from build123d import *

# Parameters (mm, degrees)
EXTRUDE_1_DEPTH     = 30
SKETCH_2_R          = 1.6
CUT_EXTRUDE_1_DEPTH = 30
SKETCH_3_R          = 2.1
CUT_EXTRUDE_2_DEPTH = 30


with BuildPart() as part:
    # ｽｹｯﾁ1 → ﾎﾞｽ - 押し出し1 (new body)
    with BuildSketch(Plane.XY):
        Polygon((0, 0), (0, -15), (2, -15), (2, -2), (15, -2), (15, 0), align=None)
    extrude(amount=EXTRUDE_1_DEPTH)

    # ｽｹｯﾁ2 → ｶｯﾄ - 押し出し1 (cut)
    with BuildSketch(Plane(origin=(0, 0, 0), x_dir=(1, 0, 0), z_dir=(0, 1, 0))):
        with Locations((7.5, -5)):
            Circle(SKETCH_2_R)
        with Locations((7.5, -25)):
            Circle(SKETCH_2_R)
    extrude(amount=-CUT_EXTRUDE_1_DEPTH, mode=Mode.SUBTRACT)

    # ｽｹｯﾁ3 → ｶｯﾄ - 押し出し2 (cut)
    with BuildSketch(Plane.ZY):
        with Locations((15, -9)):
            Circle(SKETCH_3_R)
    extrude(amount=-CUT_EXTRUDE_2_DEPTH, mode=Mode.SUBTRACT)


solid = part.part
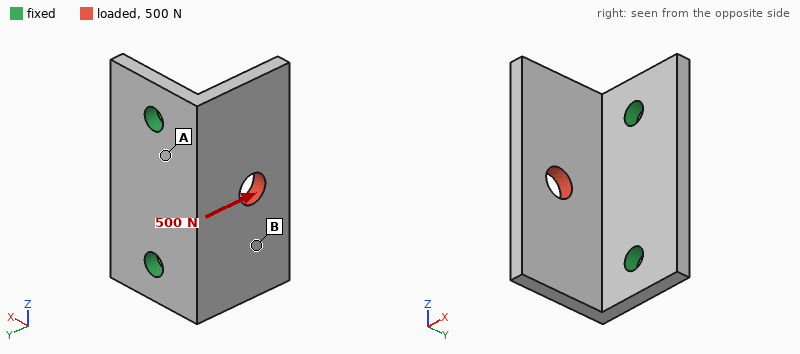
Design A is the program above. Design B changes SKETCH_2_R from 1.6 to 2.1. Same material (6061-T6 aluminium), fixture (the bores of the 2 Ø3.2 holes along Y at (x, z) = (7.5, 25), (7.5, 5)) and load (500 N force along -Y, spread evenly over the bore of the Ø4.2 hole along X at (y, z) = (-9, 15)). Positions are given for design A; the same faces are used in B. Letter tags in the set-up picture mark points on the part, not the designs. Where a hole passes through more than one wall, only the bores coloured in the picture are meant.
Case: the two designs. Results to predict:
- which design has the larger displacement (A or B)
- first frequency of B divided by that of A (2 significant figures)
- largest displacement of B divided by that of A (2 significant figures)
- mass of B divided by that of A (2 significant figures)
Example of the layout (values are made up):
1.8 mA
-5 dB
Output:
A
1.1
0.80
0.99
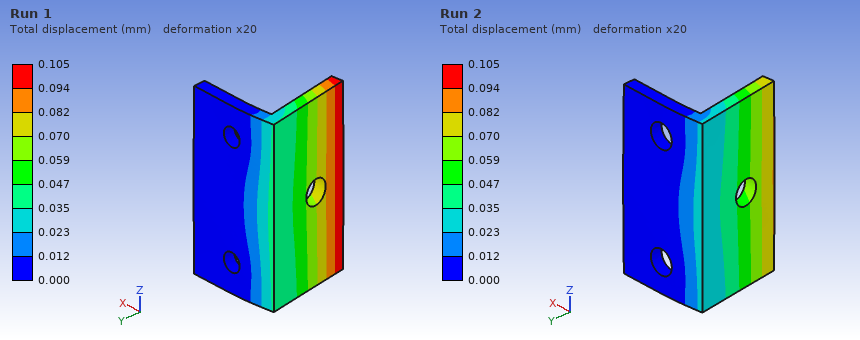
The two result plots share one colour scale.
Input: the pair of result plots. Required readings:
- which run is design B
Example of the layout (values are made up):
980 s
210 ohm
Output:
Run 2
